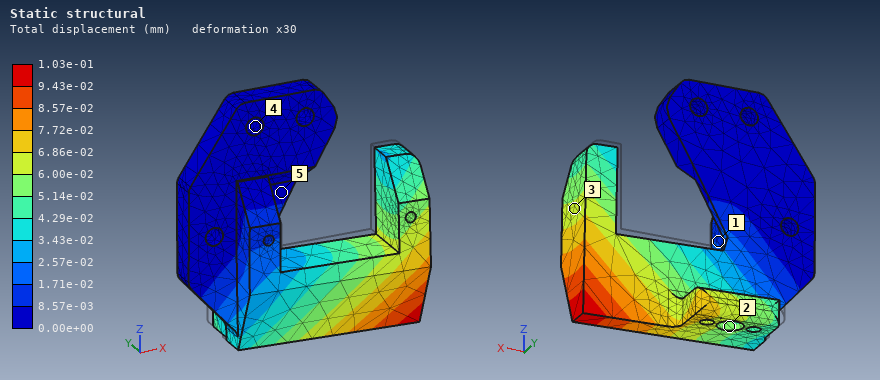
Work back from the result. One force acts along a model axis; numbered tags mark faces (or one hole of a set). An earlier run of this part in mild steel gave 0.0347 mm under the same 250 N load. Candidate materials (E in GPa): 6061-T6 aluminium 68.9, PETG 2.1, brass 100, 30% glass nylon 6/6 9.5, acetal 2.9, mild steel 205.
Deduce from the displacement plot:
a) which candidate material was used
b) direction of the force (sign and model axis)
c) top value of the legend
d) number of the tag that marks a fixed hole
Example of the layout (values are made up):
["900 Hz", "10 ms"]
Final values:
["6061-T6 aluminium", "-Y", "1.03e-01 mm", "4"]
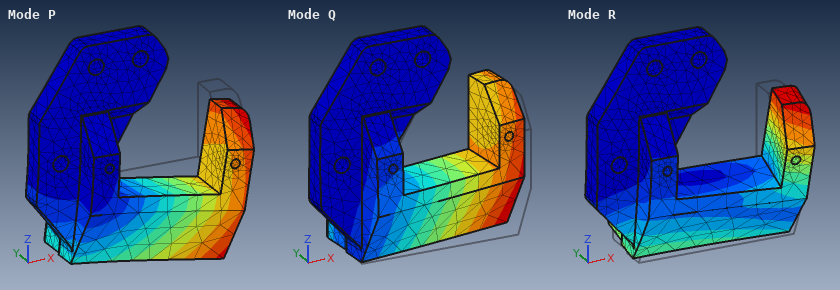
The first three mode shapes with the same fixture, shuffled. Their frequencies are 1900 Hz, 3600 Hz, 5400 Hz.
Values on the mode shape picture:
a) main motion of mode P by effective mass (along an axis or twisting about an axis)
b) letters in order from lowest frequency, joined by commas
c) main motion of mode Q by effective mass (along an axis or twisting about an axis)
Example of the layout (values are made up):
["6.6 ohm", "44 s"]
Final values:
["along Z", "Q, P, R", "along Y"]
